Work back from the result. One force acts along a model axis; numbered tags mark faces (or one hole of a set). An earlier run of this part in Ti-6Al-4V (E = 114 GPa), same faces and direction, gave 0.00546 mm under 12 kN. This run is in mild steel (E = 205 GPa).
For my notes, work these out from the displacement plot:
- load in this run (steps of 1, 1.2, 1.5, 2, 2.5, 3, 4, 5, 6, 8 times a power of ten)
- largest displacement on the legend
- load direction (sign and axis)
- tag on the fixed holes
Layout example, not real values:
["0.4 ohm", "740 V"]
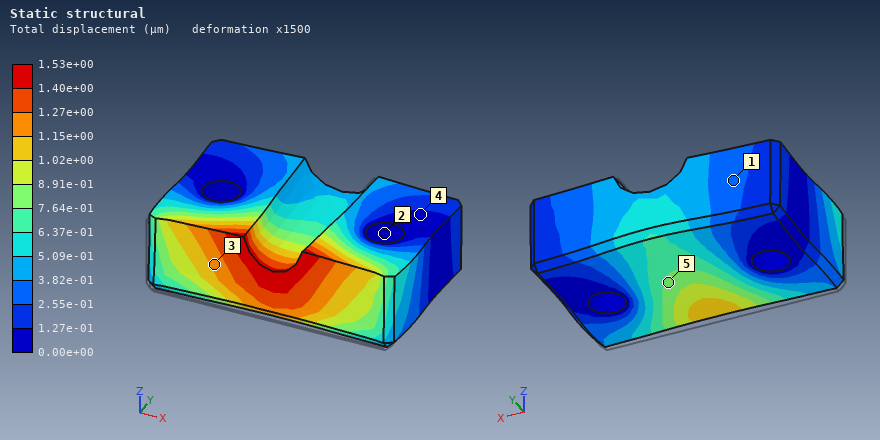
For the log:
["6 kN", "1.53e+00 µm", "+Y", "2"]
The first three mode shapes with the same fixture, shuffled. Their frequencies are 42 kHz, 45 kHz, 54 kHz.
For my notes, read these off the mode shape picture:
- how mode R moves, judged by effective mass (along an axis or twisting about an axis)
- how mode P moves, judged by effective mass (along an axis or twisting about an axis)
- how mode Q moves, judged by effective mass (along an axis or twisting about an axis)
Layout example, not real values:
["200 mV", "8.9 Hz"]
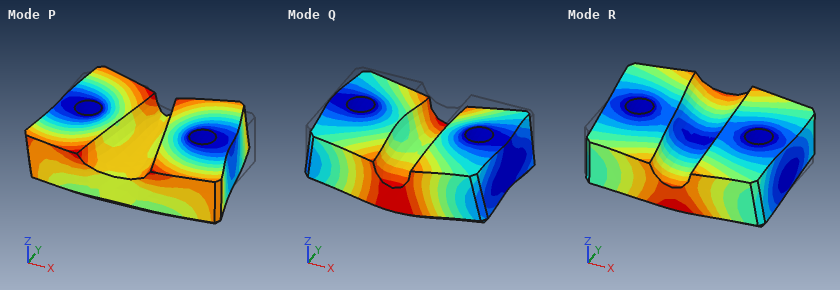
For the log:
["twisting about X", "along Y", "along Z"]
